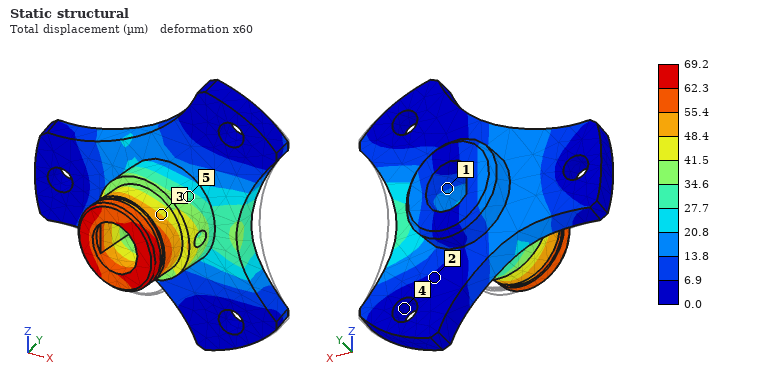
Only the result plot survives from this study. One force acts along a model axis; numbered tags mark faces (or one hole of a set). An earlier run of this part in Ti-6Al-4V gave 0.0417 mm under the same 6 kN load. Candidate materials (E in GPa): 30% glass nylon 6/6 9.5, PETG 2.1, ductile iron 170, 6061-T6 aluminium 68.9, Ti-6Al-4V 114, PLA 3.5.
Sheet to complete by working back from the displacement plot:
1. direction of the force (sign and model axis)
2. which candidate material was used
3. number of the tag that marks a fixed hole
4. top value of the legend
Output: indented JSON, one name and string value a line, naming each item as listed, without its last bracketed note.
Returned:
{
  "direction of the force": "-X",
  "which candidate material was used": "6061-T6 aluminium",
  "number of the tag that marks a fixed hole": "4",
  "top value of the legend": "69.2 µm"
}
